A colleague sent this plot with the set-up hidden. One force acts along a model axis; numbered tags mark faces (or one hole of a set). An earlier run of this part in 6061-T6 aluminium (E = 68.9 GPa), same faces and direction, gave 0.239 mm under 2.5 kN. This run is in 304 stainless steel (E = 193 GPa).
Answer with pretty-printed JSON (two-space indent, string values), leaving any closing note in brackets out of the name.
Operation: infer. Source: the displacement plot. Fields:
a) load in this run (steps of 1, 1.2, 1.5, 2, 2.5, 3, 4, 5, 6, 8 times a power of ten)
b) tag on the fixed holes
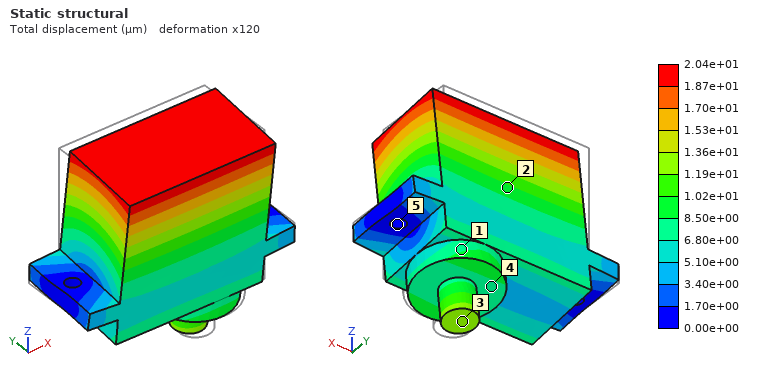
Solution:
{
  "load in this run": "600 N",
  "tag on the fixed holes": "5"
}
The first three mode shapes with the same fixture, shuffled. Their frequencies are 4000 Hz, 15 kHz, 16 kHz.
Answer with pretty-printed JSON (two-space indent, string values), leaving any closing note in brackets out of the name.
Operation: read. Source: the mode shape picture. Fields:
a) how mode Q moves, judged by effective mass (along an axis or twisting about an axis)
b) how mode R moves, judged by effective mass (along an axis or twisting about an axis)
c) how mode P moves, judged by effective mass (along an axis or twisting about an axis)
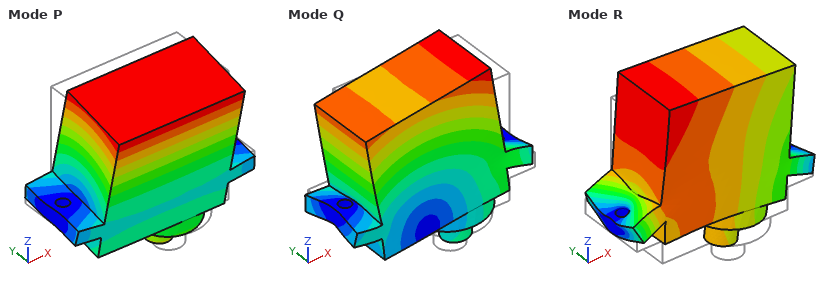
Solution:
{
  "how mode Q moves, judged by effective mass": "along X",
  "how mode R moves, judged by effective mass": "along Z",
  "how mode P moves, judged by effective mass": "along Y"
}
